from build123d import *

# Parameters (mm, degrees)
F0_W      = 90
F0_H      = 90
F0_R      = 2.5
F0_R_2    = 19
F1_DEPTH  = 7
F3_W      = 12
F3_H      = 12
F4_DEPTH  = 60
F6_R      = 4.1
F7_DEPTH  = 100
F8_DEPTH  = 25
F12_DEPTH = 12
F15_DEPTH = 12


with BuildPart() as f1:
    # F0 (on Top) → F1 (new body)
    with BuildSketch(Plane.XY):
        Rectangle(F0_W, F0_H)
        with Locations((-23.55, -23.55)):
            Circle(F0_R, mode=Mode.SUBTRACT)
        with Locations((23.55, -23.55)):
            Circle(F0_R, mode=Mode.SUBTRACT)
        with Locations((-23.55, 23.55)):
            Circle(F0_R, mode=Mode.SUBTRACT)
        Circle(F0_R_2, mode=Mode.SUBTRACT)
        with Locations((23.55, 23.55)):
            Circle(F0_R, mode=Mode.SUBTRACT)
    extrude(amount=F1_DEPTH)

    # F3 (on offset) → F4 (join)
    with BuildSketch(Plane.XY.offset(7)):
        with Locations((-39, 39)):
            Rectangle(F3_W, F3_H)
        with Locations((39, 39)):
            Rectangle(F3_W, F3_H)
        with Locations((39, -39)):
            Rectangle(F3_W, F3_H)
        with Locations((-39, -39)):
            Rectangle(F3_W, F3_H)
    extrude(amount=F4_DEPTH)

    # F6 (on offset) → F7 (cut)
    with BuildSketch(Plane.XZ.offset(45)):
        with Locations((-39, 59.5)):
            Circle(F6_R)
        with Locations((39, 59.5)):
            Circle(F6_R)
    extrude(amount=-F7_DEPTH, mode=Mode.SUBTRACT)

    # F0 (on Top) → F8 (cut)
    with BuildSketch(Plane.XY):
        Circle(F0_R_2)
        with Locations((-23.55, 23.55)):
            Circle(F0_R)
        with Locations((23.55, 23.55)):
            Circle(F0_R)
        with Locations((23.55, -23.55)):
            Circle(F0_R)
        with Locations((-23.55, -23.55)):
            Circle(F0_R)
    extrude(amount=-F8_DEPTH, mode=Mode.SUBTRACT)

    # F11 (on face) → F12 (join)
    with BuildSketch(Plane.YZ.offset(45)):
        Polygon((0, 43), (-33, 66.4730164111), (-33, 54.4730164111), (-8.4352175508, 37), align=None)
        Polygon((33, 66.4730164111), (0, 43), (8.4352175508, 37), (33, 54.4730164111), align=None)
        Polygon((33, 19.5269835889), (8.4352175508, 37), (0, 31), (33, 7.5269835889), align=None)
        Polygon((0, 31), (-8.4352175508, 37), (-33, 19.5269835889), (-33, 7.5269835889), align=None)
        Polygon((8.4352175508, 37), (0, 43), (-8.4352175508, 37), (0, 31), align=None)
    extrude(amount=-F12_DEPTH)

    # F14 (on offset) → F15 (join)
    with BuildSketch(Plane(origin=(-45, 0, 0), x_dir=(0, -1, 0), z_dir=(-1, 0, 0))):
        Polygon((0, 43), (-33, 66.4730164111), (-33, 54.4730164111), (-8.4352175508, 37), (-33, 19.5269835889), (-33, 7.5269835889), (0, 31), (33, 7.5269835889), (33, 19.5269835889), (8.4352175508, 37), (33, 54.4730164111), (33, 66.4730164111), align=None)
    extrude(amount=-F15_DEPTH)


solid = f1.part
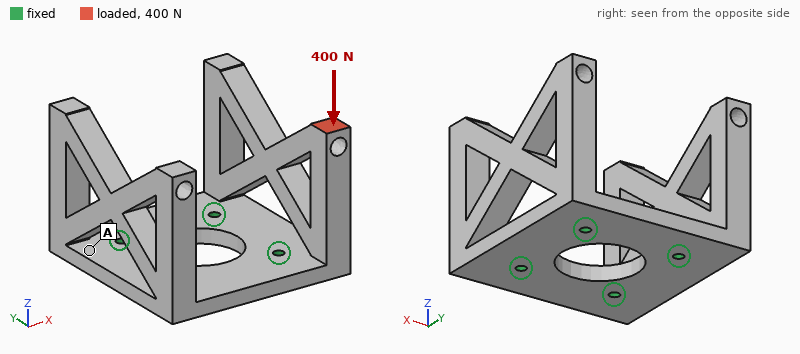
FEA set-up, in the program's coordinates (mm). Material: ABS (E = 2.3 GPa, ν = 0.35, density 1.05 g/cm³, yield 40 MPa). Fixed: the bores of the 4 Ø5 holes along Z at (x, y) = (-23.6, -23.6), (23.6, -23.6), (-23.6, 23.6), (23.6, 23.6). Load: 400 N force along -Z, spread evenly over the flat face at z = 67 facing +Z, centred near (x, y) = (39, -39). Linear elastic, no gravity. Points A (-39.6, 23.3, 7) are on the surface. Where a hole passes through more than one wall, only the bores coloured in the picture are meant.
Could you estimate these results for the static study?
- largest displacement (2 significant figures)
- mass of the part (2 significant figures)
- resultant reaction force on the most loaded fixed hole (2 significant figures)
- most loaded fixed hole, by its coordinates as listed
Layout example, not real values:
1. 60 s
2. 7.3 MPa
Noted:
1. 1.5 mm
2. 120 g
3. 490 N
4. (23.6, -23.6)
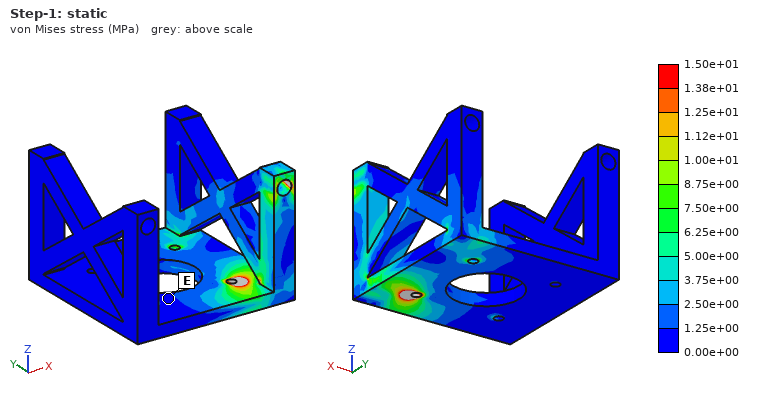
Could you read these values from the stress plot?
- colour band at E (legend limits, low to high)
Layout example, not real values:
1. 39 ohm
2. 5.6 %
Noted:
1. 0.00e+00 to 1.25e+00 MPa
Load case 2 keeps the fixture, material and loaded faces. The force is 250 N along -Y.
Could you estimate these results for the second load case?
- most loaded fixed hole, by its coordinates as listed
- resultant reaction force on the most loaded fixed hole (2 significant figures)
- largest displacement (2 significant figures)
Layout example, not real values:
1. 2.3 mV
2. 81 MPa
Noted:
1. (23.6, 23.6)
2. 320 N
3. 0.83 mm
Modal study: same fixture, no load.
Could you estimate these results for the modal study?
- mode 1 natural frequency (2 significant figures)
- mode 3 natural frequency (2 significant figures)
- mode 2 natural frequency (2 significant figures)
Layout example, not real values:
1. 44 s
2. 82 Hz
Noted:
1. 300 Hz
2. 640 Hz
3. 300 Hz
